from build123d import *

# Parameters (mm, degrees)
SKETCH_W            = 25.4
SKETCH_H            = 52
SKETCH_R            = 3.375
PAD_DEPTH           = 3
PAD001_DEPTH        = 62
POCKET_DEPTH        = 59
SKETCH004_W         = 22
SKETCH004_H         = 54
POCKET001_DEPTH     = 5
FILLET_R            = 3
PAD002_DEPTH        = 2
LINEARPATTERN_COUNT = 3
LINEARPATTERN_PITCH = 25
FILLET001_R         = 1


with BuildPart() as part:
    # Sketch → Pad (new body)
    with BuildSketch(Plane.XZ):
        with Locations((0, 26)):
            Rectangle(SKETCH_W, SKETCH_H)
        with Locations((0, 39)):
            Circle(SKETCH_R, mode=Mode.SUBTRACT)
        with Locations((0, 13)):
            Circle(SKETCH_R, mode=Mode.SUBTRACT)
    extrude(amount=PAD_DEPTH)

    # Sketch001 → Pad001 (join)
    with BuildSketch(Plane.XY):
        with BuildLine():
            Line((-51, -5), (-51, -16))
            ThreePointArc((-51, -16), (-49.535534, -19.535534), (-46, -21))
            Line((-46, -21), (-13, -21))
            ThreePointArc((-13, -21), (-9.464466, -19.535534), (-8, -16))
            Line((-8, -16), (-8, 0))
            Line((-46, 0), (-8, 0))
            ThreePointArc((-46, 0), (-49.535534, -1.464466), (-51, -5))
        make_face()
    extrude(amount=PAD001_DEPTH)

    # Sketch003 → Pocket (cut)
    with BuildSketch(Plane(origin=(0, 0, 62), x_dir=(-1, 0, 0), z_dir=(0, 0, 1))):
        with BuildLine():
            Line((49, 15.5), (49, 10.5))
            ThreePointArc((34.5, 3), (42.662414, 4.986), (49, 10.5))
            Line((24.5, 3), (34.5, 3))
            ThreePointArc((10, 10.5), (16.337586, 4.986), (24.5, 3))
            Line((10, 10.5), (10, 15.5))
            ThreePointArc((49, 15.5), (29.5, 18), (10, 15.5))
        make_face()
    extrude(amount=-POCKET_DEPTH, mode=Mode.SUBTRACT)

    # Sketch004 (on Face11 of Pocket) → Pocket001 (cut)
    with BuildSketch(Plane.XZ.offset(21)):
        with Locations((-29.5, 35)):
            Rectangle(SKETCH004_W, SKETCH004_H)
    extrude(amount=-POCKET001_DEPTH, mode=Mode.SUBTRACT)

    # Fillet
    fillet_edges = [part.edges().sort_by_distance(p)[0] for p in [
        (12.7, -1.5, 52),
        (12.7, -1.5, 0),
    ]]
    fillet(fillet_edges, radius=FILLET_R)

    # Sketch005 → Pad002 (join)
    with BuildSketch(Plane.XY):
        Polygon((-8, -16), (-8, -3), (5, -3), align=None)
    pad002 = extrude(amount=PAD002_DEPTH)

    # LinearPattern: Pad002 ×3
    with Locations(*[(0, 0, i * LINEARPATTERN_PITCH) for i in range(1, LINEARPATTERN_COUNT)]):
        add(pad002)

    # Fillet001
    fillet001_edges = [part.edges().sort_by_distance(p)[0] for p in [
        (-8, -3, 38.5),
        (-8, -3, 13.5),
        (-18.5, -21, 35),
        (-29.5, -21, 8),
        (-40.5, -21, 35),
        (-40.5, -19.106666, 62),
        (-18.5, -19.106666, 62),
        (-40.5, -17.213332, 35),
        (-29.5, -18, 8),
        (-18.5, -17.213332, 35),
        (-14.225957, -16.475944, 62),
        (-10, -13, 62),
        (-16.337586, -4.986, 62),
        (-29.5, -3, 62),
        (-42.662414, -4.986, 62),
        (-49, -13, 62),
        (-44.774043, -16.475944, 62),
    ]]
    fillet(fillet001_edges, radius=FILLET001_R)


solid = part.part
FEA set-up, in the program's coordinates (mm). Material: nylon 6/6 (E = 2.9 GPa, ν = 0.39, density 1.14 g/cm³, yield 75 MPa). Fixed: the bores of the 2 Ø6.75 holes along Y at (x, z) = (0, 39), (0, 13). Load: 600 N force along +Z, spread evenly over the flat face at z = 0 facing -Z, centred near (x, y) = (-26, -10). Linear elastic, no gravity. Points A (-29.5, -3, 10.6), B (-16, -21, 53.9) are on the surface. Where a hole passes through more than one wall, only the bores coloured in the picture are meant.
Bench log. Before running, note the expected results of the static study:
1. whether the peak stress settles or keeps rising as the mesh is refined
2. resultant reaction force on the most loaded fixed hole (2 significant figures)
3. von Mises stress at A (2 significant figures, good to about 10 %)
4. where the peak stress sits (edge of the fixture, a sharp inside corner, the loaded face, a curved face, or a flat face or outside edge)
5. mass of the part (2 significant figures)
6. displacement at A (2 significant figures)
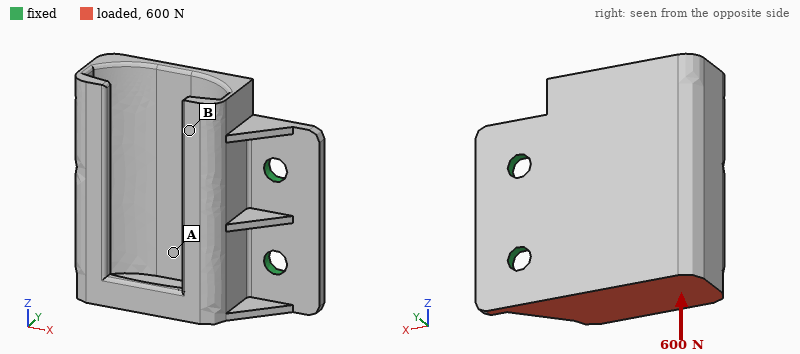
keeps rising
610 N
6.0 MPa
a sharp inside corner
29 g
0.18 mm
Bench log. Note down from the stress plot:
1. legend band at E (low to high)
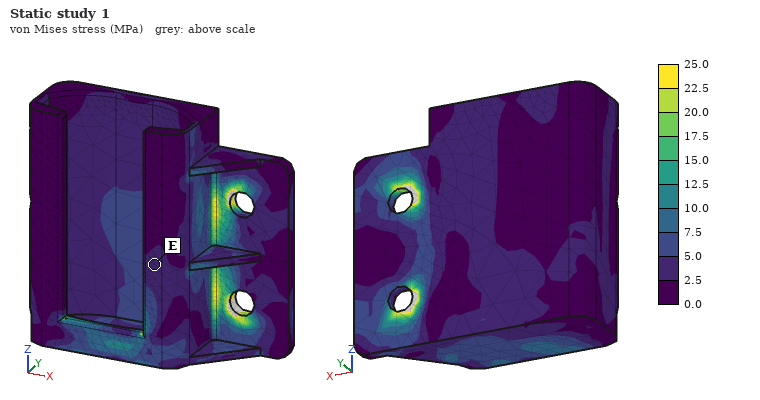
2.5 to 5.0 MPa
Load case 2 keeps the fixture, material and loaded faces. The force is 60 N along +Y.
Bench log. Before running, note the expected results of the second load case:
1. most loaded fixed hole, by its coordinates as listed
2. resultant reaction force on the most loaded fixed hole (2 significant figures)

(0, 13)
81 N
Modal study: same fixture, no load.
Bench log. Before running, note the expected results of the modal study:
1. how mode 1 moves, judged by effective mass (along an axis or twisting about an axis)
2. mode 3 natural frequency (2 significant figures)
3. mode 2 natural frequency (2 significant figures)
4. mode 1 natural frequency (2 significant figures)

along Y
1300 Hz
750 Hz
300 Hz
